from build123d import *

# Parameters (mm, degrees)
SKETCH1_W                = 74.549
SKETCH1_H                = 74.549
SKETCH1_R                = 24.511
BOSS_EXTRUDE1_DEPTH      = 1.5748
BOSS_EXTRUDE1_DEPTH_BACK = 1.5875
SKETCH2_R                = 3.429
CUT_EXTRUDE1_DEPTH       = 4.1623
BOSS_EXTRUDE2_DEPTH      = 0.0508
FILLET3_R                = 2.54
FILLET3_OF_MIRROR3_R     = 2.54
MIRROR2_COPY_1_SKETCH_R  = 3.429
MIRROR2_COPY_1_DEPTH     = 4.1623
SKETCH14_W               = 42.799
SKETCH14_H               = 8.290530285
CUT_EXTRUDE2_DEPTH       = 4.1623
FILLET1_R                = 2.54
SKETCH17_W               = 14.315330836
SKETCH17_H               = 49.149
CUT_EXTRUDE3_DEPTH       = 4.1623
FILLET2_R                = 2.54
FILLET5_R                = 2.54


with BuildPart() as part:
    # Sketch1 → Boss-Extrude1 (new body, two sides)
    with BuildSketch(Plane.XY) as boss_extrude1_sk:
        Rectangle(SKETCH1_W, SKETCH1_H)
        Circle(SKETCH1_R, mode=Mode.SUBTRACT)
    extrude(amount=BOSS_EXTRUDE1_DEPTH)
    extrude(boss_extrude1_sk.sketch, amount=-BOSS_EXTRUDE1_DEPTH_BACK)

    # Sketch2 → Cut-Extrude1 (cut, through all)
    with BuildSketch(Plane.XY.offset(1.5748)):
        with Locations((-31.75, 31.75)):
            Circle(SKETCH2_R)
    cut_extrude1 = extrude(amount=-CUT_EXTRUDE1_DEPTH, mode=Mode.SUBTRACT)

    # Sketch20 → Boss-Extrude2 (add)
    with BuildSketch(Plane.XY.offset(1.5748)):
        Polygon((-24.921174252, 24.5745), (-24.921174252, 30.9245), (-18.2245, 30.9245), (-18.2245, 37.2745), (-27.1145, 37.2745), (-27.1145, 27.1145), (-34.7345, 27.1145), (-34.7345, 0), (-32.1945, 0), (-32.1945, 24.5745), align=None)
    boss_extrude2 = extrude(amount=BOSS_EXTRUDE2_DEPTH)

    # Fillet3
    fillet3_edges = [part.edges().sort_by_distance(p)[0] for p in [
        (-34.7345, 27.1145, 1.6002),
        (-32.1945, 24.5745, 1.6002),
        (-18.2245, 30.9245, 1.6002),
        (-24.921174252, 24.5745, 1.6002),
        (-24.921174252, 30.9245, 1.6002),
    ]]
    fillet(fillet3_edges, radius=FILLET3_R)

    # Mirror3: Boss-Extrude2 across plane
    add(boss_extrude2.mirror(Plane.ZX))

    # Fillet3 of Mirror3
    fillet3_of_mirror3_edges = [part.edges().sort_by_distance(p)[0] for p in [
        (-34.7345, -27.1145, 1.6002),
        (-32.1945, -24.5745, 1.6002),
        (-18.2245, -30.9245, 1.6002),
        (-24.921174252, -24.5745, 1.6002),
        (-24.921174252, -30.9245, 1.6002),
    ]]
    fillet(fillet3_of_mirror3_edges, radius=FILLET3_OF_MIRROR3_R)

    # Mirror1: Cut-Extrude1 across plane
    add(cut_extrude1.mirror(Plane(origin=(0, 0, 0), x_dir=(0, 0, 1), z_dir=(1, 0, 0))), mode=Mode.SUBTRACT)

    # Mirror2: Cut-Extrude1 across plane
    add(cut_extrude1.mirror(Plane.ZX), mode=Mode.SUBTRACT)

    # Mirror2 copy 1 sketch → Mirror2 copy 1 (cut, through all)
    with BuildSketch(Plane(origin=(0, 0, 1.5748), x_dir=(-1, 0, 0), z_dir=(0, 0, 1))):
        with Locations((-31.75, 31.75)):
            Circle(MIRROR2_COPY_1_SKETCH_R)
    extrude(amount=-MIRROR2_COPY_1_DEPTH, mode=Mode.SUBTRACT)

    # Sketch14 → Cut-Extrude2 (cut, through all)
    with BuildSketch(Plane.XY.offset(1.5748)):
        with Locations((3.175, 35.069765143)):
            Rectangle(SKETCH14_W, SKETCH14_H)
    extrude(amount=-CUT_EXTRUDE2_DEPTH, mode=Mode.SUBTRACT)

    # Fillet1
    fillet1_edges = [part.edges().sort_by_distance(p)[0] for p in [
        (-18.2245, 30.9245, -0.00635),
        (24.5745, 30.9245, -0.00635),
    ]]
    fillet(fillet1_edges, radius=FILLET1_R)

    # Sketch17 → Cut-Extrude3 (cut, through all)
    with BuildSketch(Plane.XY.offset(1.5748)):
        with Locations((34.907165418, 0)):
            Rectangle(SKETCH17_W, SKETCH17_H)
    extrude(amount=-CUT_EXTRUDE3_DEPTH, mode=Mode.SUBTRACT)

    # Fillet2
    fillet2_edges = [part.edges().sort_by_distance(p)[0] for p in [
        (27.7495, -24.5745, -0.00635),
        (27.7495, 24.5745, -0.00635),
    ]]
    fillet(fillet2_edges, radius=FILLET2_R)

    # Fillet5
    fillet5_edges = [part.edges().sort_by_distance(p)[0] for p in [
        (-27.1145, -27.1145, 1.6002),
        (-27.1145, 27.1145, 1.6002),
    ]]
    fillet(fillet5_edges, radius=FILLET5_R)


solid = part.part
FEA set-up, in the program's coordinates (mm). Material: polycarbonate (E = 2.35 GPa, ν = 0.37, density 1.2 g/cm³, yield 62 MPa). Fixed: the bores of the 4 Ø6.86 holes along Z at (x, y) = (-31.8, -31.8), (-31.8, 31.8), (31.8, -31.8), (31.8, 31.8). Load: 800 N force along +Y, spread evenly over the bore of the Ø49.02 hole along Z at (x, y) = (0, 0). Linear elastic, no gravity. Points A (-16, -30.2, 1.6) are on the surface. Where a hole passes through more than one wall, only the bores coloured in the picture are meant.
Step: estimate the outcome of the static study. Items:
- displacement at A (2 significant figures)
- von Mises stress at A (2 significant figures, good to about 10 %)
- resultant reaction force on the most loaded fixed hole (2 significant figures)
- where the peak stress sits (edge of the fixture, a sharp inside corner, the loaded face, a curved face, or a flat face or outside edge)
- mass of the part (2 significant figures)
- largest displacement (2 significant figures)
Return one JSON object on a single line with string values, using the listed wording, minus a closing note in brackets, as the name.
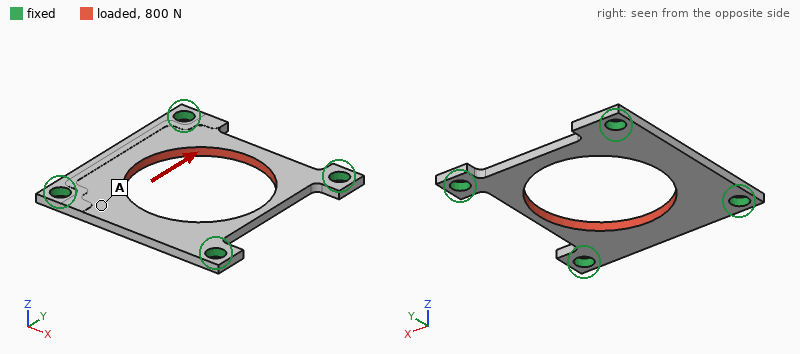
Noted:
{"displacement at A": "0.073 mm", "von Mises stress at A": "3.7 MPa", "resultant reaction force on the most loaded fixed hole": "240 N", "where the peak stress sits": "a curved face", "mass of the part": "11 g", "largest displacement": "0.32 mm"}
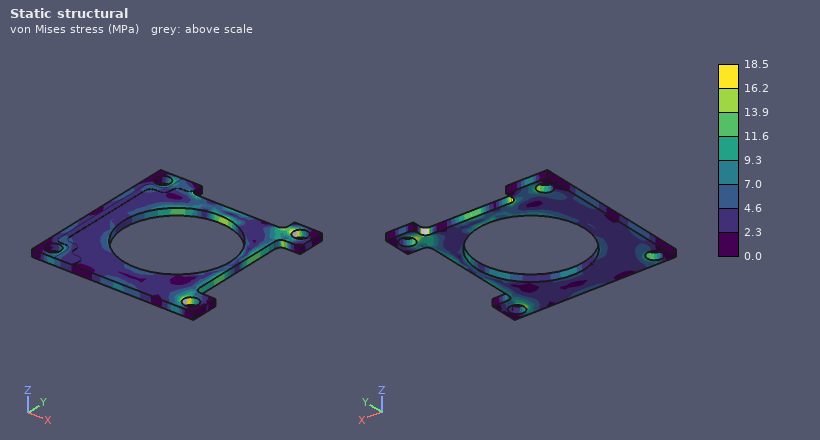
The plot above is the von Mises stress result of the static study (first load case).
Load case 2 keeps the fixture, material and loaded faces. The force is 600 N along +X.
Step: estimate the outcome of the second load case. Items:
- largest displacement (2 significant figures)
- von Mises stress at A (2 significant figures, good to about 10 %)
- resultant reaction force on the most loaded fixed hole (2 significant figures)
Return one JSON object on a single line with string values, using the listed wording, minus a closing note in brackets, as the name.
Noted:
{"largest displacement": "0.39 mm", "von Mises stress at A": "2.6 MPa", "resultant reaction force on the most loaded fixed hole": "170 N"}
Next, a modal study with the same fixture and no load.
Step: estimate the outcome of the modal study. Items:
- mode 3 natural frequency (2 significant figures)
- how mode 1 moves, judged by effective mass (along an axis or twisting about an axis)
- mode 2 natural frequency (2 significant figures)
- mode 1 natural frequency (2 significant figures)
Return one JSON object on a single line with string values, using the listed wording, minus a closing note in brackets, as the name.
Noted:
{"mode 3 natural frequency": "1400 Hz", "how mode 1 moves, judged by effective mass": "along Z", "mode 2 natural frequency": "1400 Hz", "mode 1 natural frequency": "1300 Hz"}
